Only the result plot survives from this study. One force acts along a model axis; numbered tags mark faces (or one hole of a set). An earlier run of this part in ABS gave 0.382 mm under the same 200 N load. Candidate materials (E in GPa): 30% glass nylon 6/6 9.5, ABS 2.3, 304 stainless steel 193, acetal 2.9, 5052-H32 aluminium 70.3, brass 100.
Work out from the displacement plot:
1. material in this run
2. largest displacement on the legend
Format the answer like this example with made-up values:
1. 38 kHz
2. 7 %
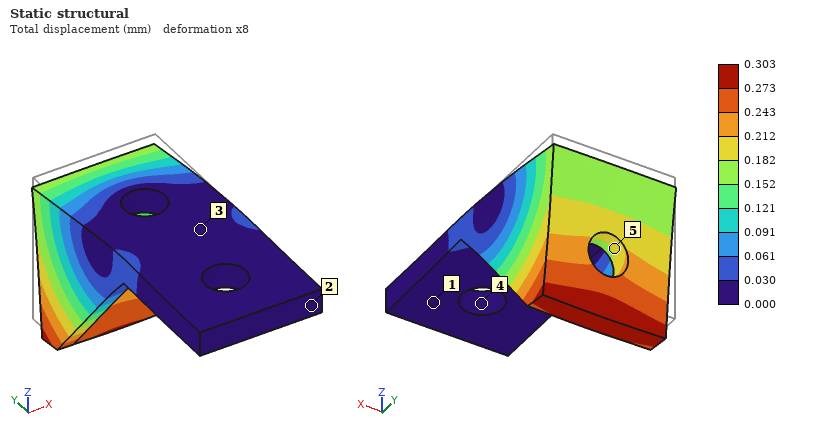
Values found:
1. acetal
2. 0.303 mm
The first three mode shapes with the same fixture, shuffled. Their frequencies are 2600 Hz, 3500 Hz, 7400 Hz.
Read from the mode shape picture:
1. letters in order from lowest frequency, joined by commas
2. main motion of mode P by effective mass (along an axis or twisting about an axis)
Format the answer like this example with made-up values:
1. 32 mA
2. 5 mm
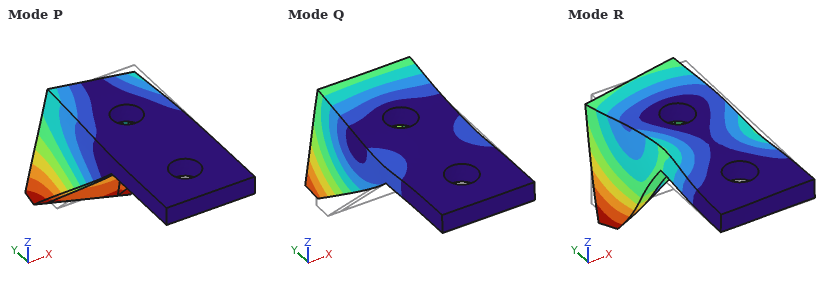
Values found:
1. P, Q, R
2. along X
